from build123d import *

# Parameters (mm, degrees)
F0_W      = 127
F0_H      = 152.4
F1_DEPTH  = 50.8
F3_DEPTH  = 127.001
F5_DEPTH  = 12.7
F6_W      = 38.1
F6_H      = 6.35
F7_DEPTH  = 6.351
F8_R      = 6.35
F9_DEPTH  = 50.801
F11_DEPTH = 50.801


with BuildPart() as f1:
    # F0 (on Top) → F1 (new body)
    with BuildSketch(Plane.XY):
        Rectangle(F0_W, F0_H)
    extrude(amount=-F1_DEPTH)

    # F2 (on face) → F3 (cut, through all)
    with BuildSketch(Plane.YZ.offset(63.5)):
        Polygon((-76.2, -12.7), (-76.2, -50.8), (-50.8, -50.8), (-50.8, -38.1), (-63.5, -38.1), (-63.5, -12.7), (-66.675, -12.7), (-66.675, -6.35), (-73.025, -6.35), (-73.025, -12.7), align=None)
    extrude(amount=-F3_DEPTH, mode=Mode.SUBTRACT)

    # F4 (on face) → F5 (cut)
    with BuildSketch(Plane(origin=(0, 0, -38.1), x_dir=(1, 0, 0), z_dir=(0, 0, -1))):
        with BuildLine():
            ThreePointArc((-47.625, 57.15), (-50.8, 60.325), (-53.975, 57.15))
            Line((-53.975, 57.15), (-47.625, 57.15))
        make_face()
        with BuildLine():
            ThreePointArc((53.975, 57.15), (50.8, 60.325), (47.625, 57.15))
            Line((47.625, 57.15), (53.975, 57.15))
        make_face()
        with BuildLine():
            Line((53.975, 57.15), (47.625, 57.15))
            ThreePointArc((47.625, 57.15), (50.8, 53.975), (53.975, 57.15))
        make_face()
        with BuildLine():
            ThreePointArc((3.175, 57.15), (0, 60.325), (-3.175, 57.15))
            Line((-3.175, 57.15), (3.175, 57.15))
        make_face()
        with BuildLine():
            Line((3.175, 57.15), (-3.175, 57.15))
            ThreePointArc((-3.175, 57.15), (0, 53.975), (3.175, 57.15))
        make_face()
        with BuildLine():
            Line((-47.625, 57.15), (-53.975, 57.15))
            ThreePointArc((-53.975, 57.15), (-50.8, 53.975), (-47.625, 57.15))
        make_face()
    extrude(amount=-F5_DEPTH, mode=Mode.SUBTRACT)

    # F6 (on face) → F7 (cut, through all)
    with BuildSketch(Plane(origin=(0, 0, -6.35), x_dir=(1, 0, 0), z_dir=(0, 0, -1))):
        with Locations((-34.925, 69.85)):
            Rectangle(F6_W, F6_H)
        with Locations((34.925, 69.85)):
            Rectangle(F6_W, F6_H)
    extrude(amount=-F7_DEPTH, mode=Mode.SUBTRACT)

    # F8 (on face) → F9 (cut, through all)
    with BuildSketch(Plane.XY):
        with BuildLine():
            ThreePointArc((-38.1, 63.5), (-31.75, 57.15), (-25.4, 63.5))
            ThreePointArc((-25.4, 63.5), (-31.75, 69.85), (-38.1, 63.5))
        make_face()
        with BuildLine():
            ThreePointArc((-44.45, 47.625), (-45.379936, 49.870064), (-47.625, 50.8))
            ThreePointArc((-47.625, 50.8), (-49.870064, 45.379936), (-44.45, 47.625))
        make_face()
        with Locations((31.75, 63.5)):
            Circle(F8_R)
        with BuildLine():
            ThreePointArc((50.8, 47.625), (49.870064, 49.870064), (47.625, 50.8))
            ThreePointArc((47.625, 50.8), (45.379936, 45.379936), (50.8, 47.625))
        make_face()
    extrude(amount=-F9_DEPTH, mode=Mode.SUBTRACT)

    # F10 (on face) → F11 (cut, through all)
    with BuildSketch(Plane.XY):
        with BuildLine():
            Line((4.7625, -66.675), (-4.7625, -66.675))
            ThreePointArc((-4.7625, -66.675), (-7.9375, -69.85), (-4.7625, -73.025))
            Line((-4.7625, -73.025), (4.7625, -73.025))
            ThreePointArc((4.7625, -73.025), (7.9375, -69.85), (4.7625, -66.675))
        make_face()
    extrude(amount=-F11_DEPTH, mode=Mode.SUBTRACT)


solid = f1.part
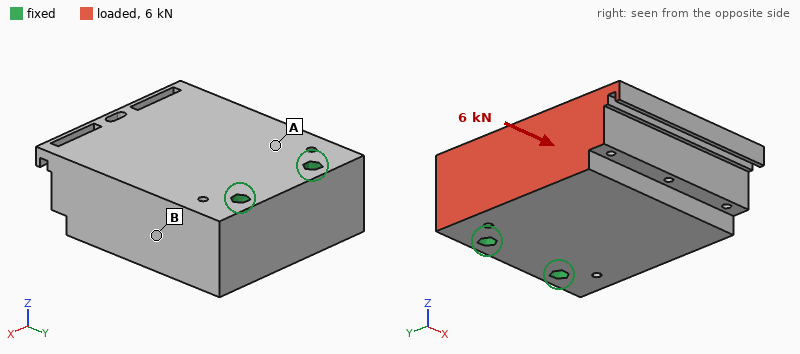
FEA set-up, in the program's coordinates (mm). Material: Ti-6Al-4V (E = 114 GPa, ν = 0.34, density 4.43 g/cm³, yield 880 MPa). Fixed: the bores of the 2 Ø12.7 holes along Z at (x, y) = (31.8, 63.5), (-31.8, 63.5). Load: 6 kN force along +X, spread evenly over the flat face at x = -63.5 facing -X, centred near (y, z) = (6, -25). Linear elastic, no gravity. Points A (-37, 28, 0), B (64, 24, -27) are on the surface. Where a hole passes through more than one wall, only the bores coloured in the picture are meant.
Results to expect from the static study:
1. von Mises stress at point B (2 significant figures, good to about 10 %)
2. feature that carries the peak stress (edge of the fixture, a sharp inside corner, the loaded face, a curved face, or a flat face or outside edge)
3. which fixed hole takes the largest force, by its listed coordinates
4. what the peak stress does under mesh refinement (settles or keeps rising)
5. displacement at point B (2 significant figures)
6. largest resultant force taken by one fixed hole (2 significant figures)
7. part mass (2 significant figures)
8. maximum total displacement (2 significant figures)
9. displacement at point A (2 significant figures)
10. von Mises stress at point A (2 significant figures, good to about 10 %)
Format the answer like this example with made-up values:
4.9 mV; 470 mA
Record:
0.80 MPa; edge of the fixture; (-31.8, 63.5); keeps rising; 2.2 µm; 5.9 kN; 3.9 kg; 6.3 µm; 1.8 µm; 1.9 MPa
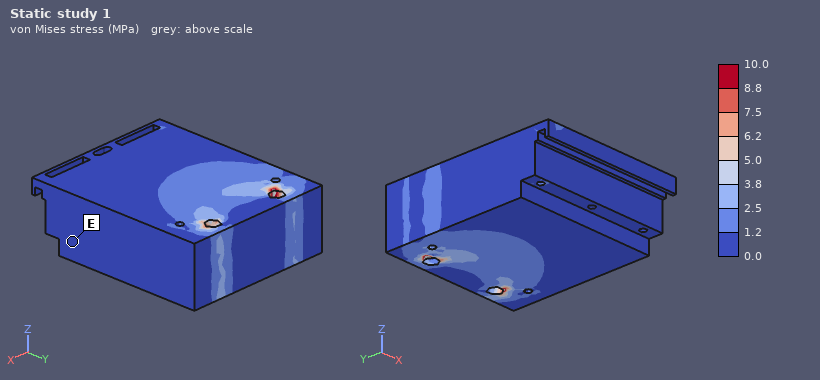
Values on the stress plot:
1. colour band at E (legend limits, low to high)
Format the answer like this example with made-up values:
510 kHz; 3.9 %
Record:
0.0 to 1.2 MPa
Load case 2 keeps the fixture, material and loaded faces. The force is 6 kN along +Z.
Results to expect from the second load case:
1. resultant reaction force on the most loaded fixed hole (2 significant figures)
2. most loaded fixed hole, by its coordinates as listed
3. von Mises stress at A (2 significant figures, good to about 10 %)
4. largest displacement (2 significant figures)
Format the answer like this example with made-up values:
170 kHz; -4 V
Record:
6.5 kN; (-31.8, 63.5); 5.4 MPa; 25 µm
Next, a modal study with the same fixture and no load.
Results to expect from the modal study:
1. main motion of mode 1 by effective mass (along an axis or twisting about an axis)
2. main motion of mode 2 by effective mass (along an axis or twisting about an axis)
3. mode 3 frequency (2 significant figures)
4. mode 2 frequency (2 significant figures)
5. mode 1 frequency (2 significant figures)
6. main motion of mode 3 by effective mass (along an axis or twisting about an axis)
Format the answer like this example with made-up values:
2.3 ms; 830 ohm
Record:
along Z; along X; 4200 Hz; 3300 Hz; 2100 Hz; twisting about Y
